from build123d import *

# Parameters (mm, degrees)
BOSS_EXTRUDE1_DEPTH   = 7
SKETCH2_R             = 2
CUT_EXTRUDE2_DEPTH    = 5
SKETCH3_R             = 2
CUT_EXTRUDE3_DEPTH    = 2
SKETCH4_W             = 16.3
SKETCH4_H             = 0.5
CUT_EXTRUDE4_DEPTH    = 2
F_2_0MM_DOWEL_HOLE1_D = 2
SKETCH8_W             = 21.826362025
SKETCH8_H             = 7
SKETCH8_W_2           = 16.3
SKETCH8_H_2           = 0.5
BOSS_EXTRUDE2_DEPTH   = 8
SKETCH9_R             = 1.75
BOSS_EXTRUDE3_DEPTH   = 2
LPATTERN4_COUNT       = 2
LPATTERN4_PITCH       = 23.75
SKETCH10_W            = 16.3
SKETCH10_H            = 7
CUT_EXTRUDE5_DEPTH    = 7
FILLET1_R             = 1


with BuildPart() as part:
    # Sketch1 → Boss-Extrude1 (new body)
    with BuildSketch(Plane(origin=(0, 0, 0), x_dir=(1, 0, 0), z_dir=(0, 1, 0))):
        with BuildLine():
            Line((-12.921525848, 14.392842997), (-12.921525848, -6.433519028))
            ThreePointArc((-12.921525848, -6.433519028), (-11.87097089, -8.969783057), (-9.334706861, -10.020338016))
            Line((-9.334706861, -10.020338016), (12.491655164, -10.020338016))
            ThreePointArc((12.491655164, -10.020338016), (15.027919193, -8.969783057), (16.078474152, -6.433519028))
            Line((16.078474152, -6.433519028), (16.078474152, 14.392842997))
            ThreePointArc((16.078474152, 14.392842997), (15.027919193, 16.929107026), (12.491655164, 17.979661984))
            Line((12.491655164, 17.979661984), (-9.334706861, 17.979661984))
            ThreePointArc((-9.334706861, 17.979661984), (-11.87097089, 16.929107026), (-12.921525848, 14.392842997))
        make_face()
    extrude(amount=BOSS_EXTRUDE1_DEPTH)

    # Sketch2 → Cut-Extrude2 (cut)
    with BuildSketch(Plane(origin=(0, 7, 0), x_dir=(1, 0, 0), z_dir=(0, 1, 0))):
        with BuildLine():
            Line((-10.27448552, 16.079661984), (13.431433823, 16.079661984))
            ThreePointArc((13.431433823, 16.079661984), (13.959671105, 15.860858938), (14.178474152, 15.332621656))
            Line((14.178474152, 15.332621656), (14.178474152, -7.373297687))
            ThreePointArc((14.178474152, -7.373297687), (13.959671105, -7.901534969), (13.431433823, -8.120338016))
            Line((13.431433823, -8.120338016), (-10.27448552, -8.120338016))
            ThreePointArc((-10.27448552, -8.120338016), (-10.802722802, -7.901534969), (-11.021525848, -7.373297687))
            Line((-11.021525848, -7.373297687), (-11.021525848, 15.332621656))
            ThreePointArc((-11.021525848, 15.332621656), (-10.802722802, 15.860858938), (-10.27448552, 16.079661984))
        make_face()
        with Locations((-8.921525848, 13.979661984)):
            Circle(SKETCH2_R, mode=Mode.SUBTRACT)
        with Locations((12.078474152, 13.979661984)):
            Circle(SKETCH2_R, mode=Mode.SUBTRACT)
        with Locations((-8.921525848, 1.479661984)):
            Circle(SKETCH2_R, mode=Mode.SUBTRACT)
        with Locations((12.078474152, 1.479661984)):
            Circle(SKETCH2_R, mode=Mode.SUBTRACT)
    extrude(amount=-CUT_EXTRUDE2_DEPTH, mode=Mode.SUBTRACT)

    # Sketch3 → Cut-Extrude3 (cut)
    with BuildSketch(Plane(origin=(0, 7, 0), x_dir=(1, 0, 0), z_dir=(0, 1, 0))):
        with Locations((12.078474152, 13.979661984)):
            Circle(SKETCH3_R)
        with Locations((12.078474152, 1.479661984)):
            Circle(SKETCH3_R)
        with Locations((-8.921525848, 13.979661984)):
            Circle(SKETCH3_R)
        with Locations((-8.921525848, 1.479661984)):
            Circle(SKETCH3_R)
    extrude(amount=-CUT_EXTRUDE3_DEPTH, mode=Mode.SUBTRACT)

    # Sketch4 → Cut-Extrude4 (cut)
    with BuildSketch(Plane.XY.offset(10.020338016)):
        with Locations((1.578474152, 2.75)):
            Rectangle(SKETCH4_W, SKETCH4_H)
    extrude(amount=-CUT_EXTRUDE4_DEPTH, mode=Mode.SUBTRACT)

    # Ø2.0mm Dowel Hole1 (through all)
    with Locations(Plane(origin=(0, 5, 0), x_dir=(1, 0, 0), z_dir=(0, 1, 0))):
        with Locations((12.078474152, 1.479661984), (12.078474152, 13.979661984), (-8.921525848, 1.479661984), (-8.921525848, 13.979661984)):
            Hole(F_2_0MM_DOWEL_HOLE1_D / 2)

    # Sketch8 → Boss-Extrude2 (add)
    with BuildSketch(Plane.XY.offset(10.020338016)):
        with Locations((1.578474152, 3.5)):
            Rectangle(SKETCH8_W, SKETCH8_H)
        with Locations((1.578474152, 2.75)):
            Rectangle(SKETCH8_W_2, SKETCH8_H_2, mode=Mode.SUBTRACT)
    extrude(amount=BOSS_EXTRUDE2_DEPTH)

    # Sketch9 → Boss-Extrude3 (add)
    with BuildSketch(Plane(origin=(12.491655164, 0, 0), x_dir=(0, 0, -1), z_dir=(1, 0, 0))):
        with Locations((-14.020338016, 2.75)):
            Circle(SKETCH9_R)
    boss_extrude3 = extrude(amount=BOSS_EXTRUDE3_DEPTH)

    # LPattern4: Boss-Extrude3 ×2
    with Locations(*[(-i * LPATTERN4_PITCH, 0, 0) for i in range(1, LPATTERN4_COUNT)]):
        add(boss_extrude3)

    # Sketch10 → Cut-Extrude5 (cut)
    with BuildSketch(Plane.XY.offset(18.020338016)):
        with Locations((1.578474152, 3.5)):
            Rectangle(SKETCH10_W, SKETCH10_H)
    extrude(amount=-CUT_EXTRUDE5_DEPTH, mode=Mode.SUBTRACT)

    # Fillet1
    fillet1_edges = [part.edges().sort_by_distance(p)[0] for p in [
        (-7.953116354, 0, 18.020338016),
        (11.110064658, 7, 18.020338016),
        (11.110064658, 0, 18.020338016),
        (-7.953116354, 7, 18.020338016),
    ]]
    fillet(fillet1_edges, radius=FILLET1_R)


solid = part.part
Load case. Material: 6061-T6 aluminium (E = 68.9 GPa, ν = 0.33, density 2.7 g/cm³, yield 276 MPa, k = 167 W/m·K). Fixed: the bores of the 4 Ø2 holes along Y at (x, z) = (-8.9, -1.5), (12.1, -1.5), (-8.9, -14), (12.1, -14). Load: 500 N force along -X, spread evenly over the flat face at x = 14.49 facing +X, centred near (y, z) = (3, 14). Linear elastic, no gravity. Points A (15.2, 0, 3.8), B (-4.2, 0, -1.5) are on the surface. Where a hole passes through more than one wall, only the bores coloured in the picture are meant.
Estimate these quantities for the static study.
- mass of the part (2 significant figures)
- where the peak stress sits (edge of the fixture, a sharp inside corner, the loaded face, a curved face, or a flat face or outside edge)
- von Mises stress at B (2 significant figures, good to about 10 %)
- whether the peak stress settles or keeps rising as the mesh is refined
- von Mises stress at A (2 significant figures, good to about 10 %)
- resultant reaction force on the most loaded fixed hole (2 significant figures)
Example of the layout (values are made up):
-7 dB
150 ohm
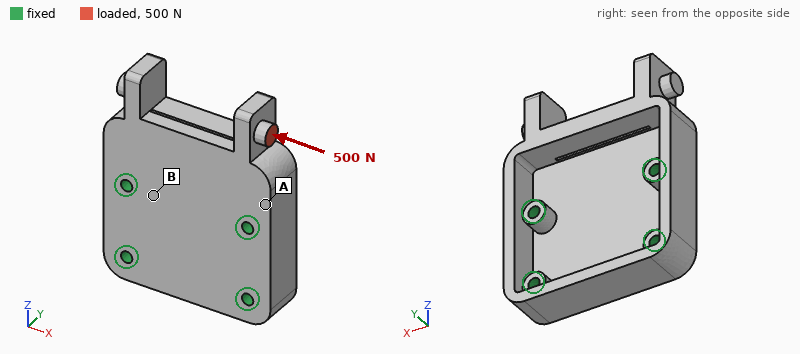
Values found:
8.3 g
a sharp inside corner
15 MPa
keeps rising
33 MPa
400 N
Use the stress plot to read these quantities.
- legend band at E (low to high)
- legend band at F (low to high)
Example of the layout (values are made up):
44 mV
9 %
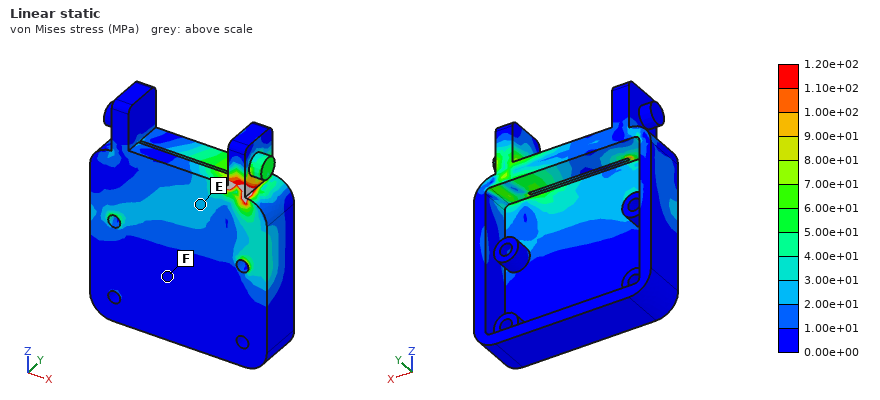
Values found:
2.00e+01 to 3.00e+01 MPa
0.00e+00 to 1.00e+01 MPa
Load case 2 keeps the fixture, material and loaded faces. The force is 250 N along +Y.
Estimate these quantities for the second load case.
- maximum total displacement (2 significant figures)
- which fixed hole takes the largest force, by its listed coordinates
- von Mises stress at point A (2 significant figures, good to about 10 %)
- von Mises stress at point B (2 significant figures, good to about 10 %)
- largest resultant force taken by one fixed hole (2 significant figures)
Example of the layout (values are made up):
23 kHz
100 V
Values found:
0.14 mm
(12.1, -1.5)
62 MPa
16 MPa
500 N
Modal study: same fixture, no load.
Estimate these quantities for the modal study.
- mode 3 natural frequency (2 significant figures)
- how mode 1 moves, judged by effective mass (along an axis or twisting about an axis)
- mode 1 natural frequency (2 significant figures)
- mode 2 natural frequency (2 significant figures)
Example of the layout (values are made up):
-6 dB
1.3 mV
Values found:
19 kHz
along Y
8100 Hz
11 kHz
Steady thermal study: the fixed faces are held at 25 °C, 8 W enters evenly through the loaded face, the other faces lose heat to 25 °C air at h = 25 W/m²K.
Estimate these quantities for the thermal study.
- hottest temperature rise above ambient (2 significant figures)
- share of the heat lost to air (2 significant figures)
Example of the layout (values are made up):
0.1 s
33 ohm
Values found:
37 K
4.5 %
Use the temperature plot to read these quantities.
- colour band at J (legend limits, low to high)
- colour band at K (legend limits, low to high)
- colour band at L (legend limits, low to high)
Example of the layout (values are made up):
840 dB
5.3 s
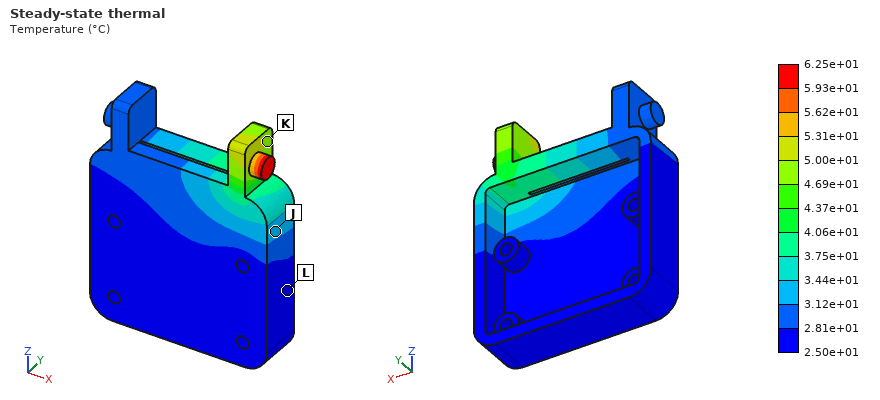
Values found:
3.12e+01 to 3.44e+01 °C
4.69e+01 to 5.00e+01 °C
2.50e+01 to 2.81e+01 °C
